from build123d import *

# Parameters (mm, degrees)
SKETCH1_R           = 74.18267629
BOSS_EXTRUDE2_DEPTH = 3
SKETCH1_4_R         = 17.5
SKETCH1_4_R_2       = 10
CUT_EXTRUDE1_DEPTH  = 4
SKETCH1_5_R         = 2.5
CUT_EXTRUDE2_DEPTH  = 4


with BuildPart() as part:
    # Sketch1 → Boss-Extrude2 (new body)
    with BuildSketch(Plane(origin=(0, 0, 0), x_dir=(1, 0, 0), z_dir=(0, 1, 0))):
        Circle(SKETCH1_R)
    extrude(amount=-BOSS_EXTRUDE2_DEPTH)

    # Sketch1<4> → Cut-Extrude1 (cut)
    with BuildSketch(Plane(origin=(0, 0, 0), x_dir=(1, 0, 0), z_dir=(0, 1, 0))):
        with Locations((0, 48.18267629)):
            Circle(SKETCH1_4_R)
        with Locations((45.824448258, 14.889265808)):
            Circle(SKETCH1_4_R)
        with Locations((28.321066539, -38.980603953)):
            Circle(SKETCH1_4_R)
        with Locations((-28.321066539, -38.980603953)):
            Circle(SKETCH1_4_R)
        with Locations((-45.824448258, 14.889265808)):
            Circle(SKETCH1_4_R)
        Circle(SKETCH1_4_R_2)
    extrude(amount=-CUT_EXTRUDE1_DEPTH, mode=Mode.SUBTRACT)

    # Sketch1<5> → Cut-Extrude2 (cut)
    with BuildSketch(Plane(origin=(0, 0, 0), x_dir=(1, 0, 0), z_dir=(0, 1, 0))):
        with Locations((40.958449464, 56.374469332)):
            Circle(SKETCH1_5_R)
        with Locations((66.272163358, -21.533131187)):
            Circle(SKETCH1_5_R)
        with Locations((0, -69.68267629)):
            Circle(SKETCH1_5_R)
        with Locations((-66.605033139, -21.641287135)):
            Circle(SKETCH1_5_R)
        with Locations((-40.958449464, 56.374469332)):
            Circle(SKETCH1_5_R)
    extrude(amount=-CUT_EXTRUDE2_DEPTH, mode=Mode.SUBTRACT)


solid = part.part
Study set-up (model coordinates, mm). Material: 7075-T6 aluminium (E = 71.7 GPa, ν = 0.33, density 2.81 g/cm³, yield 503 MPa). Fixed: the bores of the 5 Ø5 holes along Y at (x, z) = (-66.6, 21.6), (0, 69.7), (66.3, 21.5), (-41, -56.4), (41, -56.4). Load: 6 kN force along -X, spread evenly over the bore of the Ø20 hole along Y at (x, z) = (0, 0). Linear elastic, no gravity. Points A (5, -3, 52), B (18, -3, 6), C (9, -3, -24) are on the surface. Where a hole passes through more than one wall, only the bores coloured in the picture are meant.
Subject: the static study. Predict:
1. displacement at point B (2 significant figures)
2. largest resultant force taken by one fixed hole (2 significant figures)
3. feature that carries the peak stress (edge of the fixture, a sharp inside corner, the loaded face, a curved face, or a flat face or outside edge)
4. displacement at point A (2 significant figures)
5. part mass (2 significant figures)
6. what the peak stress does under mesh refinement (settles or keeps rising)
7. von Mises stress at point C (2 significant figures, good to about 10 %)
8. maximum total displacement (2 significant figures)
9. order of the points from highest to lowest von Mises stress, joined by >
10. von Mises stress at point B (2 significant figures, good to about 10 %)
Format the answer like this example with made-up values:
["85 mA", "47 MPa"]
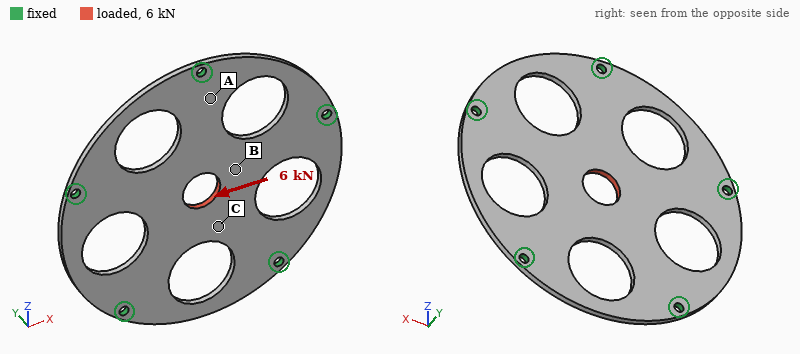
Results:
["23 µm", "1.9 kN", "edge of the fixture", "7.1 µm", "100 g", "keeps rising", "20 MPa", "28 µm", "B > C > A", "34 MPa"]
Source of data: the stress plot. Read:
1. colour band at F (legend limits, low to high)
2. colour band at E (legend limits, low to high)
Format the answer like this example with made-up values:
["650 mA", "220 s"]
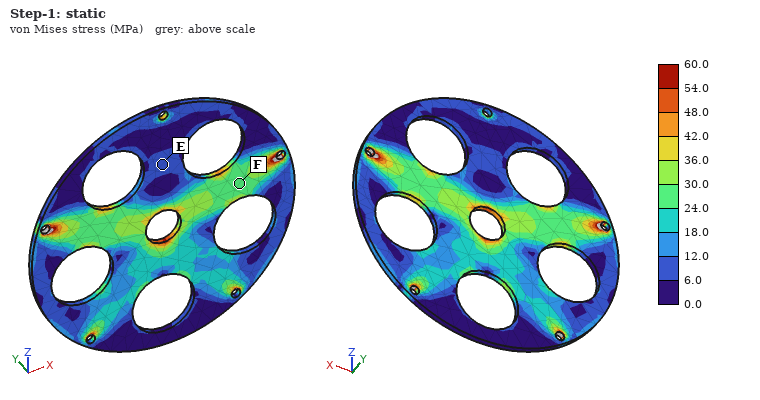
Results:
["24.0 to 30.0 MPa", "6.0 to 12.0 MPa"]
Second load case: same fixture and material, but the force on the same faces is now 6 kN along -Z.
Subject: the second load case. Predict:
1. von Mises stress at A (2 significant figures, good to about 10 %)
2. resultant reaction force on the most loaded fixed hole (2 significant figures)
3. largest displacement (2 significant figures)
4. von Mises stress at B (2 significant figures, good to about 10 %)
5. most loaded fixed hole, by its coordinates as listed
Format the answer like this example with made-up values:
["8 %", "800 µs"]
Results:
["31 MPa", "2.0 kN", "28 µm", "12 MPa", "(0, 69.7)"]
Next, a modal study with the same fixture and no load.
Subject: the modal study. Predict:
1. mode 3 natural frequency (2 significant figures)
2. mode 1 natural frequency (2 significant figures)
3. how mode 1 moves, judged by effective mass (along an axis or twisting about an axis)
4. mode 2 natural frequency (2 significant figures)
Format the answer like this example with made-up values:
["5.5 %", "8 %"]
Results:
["2400 Hz", "1100 Hz", "along Y", "2300 Hz"]
